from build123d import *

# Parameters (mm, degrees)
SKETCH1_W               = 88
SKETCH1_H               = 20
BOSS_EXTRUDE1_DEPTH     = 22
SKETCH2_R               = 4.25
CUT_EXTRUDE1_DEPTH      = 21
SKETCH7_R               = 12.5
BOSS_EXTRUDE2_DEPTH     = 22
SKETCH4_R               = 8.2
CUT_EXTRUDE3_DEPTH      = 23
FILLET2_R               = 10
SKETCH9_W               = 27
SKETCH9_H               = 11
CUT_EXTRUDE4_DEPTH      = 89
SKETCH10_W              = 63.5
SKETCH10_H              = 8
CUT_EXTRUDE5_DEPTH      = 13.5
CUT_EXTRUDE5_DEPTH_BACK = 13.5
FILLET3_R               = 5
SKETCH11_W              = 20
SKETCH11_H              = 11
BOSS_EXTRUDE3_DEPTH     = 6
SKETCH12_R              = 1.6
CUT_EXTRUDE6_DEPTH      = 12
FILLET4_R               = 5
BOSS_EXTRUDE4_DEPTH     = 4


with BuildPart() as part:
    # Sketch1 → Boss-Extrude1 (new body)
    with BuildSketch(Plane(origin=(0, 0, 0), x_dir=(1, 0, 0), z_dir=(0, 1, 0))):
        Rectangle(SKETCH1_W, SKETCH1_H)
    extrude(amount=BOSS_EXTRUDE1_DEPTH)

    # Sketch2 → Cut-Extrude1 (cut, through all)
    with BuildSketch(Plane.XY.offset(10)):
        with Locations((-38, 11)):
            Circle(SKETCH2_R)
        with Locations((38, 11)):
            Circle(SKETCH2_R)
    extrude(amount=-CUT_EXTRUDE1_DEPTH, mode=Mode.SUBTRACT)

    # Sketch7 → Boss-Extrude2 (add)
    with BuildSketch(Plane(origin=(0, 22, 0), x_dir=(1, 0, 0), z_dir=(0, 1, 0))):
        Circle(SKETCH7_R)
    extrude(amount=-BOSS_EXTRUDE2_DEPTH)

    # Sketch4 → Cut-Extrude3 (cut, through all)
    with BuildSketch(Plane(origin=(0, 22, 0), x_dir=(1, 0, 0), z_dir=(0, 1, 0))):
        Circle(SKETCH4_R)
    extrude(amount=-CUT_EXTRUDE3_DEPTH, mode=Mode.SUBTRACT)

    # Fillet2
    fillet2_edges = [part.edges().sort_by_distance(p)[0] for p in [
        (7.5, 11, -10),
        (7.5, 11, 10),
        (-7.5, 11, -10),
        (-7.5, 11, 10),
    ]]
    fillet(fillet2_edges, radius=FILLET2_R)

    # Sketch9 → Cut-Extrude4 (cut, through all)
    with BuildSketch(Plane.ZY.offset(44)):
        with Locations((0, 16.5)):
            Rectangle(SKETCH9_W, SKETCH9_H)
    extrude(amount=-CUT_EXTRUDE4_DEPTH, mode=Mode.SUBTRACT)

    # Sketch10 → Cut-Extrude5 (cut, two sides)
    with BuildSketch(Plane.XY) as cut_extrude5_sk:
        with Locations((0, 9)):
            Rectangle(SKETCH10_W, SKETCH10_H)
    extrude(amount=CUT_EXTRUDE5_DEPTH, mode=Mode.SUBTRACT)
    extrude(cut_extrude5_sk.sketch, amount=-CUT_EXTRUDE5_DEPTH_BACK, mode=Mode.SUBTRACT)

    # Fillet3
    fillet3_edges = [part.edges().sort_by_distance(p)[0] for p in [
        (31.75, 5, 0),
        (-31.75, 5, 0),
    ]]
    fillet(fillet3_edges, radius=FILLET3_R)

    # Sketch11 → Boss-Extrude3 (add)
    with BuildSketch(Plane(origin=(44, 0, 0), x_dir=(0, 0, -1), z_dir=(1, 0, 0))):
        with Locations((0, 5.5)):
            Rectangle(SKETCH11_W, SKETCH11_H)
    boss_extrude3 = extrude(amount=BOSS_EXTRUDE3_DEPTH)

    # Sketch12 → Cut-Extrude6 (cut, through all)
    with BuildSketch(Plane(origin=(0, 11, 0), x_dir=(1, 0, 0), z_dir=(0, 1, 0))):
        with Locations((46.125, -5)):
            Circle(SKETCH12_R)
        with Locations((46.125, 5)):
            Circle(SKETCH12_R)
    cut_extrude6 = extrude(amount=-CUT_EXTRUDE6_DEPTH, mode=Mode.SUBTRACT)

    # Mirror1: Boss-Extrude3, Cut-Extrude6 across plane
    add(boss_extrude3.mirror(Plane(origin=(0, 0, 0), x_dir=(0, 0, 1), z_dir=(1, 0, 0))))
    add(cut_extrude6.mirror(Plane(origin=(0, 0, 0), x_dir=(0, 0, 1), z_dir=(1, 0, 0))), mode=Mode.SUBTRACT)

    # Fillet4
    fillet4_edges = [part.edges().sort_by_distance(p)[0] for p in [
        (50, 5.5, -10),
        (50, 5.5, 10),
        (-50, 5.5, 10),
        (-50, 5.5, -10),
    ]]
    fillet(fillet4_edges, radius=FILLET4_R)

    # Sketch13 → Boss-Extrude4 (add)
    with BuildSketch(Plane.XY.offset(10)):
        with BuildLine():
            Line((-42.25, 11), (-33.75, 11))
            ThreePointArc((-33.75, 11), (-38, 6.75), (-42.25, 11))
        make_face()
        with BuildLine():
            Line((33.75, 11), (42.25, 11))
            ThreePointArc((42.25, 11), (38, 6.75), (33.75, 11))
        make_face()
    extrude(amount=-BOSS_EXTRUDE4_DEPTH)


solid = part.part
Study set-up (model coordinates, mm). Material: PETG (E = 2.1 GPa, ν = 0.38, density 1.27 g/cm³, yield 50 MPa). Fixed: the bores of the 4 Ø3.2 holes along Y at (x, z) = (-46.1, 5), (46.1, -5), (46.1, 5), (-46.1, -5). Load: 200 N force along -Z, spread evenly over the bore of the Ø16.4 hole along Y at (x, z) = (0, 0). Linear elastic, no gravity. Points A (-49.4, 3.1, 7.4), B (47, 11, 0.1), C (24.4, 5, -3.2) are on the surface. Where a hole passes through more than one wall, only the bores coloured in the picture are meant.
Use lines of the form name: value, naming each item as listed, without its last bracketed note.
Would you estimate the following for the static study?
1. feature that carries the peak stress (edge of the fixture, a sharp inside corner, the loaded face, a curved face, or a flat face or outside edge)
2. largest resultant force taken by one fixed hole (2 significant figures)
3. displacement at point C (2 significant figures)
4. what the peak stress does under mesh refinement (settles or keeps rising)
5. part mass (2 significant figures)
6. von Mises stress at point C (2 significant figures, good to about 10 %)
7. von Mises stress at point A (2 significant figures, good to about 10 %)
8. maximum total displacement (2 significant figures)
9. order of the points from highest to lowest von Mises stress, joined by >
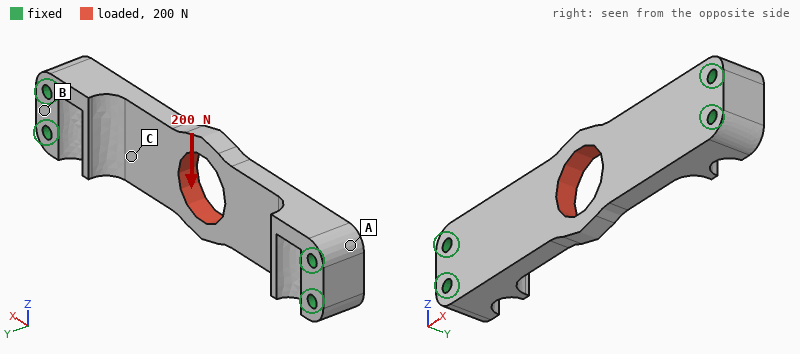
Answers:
feature that carries the peak stress: edge of the fixture
largest resultant force taken by one fixed hole: 200 N
displacement at point C: 0.069 mm
what the peak stress does under mesh refinement: keeps rising
part mass: 16 g
von Mises stress at point C: 2.6 MPa
von Mises stress at point A: 1.4 MPa
maximum total displacement: 0.15 mm
order of the points from highest to lowest von Mises stress, joined by >: C > A > B
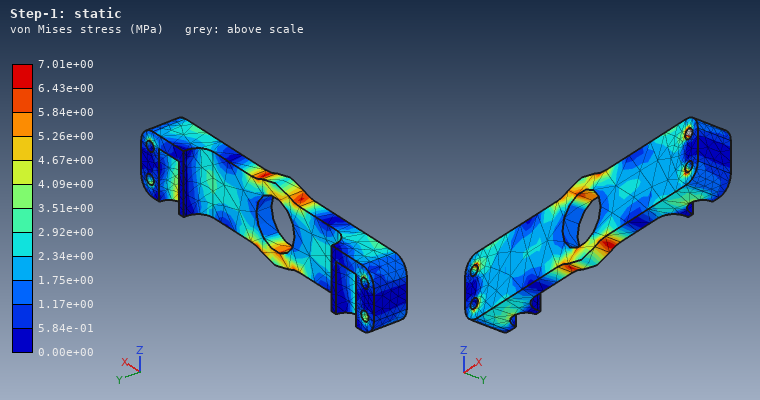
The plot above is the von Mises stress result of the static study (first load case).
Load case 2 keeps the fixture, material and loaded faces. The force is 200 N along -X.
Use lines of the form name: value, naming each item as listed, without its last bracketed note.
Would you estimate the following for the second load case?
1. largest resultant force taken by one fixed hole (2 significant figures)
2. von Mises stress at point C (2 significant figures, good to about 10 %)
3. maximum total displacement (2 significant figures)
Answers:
largest resultant force taken by one fixed hole: 51 N
von Mises stress at point C: 1.4 MPa
maximum total displacement: 23 µm
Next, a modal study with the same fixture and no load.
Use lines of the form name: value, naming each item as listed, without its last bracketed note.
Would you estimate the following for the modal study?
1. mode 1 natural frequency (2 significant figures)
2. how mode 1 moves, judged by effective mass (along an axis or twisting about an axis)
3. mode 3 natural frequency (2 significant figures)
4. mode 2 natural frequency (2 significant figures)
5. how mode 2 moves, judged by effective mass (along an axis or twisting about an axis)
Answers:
mode 1 natural frequency: 1300 Hz
how mode 1 moves, judged by effective mass: along Y
mode 3 natural frequency: 2700 Hz
mode 2 natural frequency: 2600 Hz
how mode 2 moves, judged by effective mass: twisting about X
